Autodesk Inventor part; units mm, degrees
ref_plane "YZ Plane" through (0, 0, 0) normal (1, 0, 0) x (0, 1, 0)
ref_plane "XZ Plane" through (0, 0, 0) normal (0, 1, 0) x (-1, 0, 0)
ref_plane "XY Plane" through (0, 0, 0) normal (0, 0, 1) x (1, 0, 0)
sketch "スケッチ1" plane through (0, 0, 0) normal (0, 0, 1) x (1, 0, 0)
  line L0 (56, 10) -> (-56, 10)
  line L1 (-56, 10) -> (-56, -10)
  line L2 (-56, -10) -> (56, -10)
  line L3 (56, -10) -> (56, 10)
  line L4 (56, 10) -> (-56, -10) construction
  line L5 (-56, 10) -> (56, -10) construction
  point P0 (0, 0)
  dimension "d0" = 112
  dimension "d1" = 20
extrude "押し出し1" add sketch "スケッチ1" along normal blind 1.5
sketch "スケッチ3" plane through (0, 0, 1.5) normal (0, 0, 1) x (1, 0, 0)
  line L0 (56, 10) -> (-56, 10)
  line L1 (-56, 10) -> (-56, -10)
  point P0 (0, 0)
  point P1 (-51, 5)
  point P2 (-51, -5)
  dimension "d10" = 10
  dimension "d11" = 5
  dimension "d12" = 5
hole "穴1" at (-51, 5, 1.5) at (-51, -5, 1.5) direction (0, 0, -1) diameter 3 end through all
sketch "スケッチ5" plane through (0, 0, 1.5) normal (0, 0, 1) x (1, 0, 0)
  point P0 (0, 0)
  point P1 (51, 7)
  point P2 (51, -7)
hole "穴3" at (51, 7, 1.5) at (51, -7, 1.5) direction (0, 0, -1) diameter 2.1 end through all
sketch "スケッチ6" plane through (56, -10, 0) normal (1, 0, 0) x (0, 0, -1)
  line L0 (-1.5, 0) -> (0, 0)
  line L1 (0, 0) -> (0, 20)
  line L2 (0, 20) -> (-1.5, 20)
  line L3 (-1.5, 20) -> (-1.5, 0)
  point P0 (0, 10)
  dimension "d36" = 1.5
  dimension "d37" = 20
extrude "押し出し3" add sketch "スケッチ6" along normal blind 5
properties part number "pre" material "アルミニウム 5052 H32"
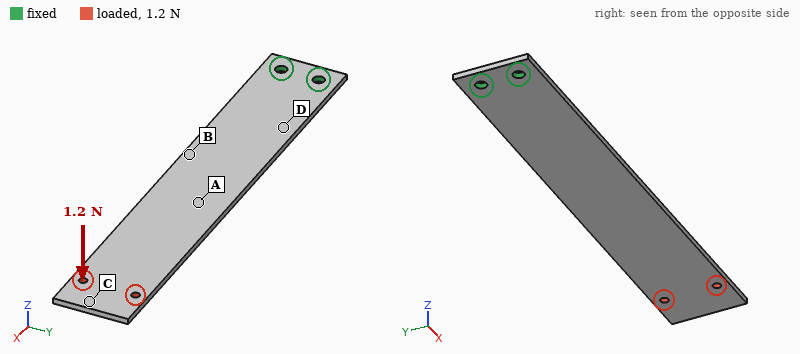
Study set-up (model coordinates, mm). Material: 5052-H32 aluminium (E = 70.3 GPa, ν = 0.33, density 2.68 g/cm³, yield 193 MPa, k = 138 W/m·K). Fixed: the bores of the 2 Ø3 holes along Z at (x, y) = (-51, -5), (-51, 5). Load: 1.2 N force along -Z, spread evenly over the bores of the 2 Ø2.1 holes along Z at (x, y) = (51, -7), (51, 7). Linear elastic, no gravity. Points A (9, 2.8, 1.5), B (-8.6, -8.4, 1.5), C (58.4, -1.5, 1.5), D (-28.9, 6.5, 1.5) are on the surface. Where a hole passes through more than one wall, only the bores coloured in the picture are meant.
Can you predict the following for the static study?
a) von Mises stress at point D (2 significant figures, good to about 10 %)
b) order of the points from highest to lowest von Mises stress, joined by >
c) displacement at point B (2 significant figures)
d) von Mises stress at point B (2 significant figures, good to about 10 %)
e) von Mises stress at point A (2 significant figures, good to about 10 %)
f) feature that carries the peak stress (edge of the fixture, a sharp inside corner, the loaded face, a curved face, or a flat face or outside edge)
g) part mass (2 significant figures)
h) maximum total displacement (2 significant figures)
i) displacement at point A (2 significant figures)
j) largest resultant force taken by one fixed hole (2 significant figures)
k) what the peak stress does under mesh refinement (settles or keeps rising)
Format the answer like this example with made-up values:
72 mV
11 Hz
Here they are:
13 MPa
D > B > A > C
0.22 mm
9.6 MPa
6.7 MPa
edge of the fixture
9.3 g
1.2 mm
0.42 mm
0.60 N
keeps rising
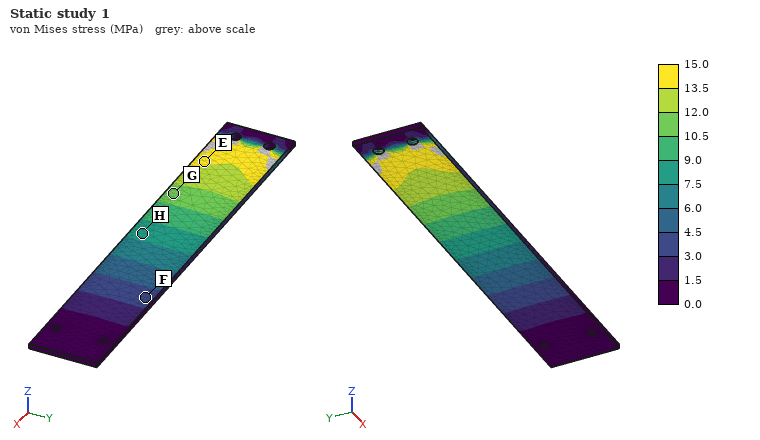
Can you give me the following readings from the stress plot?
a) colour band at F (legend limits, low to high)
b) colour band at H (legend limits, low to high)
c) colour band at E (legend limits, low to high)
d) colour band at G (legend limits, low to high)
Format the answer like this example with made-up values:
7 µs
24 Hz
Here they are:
3.0 to 4.5 MPa
7.5 to 9.0 MPa
13.5 to 15.0 MPa
10.5 to 12.0 MPa
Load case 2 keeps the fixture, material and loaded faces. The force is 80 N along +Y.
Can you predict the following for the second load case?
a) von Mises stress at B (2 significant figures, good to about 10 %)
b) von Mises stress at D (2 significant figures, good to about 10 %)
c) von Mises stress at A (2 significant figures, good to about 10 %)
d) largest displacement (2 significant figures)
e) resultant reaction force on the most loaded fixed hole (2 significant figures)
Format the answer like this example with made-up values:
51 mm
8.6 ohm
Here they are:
40 MPa
42 MPa
11 MPa
0.50 mm
690 N
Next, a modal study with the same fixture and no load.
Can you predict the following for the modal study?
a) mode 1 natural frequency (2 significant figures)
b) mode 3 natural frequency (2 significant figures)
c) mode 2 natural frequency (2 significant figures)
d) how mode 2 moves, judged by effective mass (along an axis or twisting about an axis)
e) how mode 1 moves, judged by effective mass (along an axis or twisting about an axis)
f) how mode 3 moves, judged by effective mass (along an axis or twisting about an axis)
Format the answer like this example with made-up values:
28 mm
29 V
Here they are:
100 Hz
1100 Hz
640 Hz
along Z
along Z
twisting about X
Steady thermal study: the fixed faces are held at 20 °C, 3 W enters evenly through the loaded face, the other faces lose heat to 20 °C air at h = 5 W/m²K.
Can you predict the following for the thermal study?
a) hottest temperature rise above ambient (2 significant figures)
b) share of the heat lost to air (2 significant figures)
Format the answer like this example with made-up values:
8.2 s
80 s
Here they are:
62 K
25 %
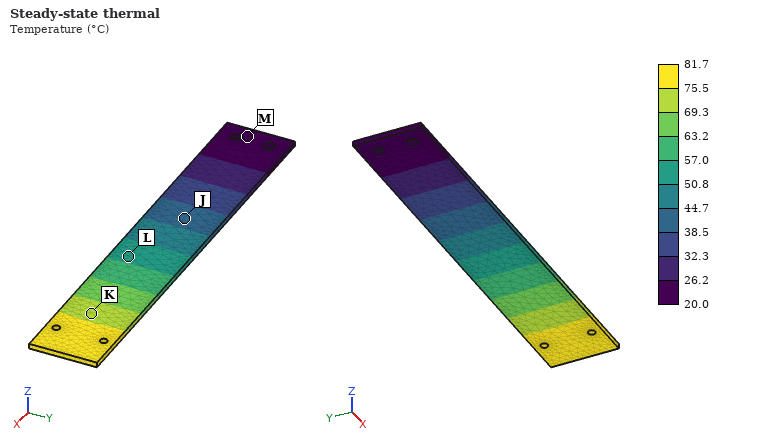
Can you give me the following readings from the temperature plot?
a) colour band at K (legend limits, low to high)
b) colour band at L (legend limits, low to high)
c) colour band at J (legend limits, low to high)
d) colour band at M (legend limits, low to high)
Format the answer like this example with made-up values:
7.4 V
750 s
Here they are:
69.3 to 75.5 °C
50.8 to 57.0 °C
38.5 to 44.7 °C
20.0 to 26.2 °C
